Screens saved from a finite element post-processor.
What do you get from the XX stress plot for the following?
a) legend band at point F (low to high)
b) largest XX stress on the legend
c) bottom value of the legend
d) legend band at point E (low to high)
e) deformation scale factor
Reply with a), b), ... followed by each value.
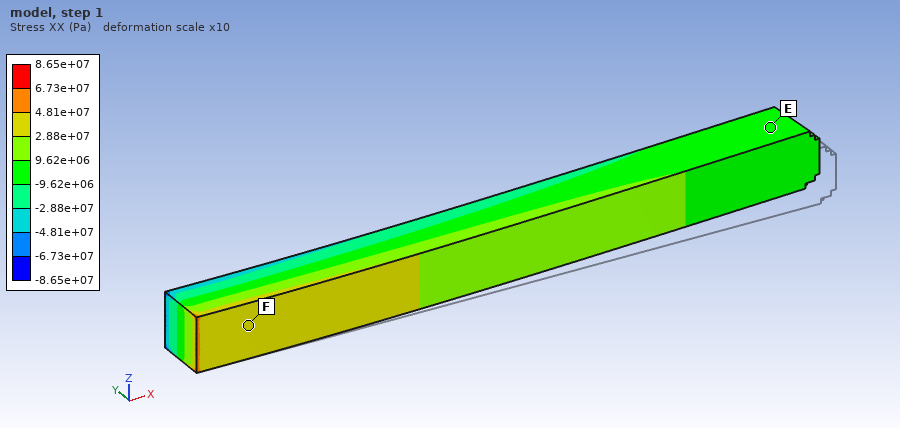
a) 2.88e+07 to 4.81e+07 Pa
b) 8.65e+07 Pa
c) -8.65e+07 Pa
d) -9.62e+06 to 9.62e+06 Pa
e) 10
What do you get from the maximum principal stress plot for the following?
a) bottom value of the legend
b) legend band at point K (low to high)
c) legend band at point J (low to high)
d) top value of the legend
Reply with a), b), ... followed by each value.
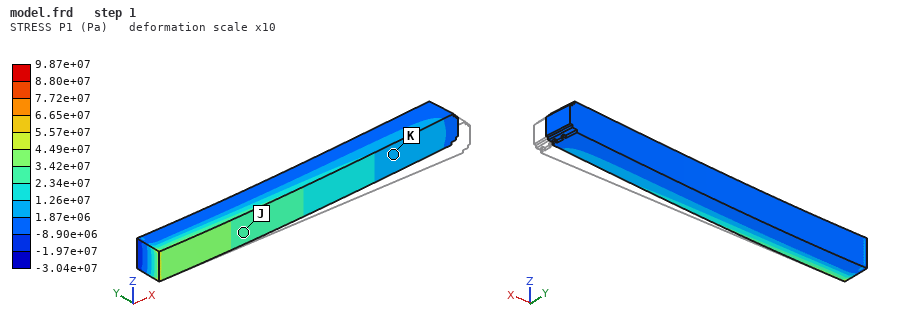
a) -3.04e+07 Pa
b) 1.87e+06 to 1.26e+07 Pa
c) 2.34e+07 to 3.42e+07 Pa
d) 9.87e+07 Pa
